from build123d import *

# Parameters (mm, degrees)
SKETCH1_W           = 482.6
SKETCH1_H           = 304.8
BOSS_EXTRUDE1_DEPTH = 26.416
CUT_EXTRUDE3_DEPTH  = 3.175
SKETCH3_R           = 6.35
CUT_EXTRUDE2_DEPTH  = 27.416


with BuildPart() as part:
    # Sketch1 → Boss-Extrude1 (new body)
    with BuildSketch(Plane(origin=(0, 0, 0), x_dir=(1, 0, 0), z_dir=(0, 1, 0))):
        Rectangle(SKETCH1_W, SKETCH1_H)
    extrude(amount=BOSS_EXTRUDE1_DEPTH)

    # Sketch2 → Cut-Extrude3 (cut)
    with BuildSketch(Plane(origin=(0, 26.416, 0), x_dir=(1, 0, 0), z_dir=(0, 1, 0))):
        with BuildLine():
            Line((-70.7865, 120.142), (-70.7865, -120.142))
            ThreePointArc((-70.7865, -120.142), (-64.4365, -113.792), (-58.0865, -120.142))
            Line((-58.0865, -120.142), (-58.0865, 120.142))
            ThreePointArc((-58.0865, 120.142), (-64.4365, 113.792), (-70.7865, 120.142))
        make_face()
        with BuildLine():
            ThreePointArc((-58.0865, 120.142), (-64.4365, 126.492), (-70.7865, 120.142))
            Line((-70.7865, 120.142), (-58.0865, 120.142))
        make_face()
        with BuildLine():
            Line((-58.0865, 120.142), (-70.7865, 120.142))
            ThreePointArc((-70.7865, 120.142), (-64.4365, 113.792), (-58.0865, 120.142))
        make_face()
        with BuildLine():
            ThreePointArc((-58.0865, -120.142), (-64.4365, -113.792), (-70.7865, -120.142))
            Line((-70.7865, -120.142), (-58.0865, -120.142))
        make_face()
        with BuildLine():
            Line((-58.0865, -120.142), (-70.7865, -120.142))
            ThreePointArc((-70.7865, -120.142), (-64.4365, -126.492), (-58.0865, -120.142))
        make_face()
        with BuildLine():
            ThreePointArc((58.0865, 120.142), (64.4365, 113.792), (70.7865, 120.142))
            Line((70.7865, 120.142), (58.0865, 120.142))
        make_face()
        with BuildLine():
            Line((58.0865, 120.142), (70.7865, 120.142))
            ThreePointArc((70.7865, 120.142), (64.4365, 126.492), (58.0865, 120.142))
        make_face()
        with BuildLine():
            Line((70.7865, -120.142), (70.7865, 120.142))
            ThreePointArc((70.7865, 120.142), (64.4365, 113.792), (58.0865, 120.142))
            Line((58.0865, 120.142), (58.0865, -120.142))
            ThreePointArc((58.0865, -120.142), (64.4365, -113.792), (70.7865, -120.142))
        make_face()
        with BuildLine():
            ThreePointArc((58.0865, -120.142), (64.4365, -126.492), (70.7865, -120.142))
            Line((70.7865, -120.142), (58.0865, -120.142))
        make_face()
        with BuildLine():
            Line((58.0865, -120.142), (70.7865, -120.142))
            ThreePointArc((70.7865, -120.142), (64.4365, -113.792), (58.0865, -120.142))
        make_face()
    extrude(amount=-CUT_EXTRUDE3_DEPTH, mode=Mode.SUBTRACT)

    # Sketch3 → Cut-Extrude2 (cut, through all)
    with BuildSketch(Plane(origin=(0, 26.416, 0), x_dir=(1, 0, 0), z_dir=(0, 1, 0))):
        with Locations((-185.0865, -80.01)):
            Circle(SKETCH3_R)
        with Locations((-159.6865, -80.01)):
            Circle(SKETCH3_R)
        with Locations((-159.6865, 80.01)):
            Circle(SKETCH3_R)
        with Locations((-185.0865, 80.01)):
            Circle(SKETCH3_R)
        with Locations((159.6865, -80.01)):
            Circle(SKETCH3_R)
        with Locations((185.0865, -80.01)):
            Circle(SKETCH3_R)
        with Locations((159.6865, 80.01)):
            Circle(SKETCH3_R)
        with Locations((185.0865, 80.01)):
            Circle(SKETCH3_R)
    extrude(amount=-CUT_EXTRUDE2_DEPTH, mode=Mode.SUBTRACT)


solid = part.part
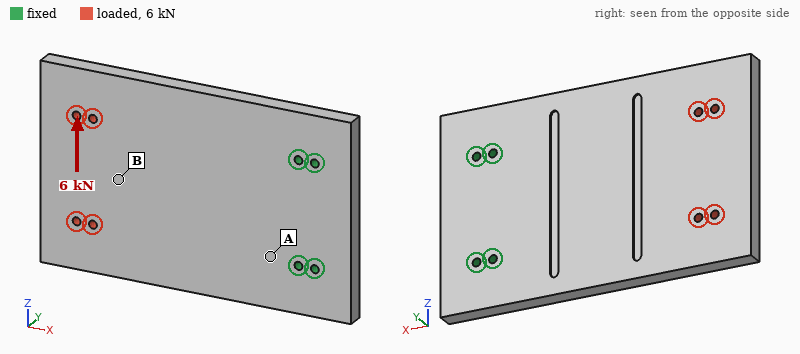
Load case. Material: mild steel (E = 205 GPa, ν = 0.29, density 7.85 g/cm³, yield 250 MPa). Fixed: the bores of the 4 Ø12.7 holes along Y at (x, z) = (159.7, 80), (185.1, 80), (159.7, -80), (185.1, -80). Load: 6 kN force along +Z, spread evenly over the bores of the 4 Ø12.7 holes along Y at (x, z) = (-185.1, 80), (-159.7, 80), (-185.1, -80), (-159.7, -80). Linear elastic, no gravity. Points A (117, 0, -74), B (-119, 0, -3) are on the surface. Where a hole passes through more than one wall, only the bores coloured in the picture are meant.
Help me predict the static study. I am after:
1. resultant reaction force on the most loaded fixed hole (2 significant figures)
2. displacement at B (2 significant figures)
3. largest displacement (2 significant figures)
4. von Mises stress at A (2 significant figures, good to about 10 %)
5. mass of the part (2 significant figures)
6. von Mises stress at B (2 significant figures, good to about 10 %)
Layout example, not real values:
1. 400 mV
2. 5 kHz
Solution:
1. 8.4 kN
2. 11 µm
3. 18 µm
4. 4.2 MPa
5. 30 kg
6. 1.8 MPa
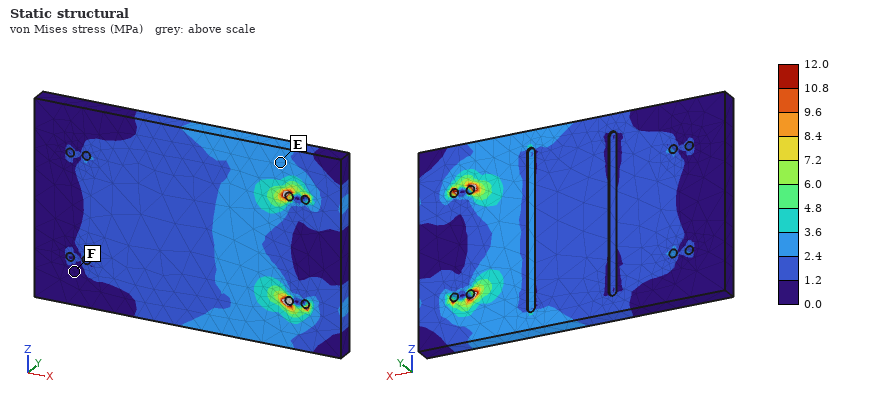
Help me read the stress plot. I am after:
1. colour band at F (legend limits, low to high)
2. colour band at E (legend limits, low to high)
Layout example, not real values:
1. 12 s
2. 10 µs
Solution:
1. 0.0 to 1.2 MPa
2. 2.4 to 3.6 MPa
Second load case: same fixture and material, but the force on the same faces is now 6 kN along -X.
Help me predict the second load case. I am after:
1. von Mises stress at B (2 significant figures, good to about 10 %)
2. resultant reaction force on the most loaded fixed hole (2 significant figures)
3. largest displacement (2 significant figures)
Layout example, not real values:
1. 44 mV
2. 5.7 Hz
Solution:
1. 0.56 MPa
2. 1.9 kN
3. 1.9 µm
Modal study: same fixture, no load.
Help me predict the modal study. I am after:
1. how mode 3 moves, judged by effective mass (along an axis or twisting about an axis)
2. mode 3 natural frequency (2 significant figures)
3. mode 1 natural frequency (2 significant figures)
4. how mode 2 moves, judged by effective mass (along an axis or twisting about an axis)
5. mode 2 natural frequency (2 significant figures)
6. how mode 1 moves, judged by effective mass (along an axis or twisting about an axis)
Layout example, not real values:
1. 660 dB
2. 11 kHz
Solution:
1. along Y
2. 770 Hz
3. 130 Hz
4. twisting about X
5. 380 Hz
6. along Y
